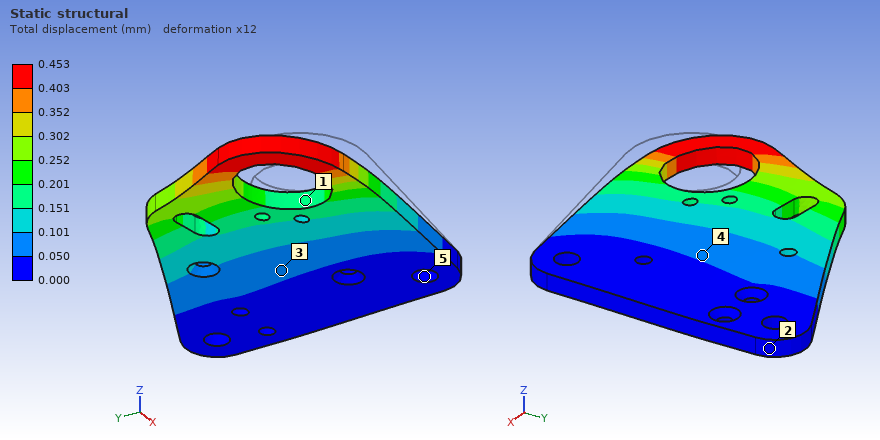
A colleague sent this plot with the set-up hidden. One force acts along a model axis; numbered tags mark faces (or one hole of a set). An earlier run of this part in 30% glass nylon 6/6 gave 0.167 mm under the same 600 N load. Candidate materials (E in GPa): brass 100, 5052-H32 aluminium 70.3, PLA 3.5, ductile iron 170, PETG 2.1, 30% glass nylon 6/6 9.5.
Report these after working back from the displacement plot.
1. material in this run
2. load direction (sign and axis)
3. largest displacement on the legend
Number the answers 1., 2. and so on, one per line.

1. PLA
2. +Y
3. 0.453 mm
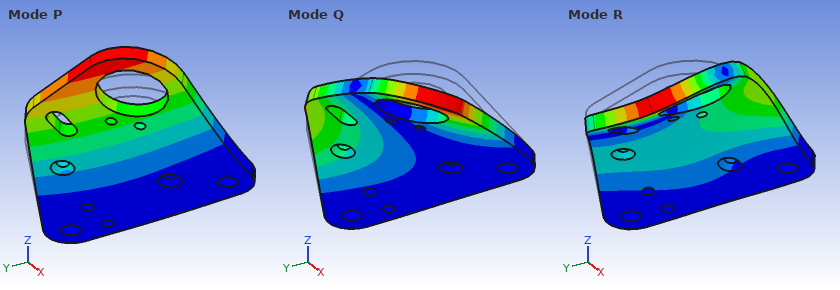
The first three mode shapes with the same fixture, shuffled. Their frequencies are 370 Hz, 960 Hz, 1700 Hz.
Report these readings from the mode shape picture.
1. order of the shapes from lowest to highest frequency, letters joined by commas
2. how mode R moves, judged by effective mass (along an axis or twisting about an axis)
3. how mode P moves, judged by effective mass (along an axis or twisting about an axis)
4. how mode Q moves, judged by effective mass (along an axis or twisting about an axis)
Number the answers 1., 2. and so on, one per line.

1. P, Q, R
2. along Z
3. along Z
4. twisting about X
